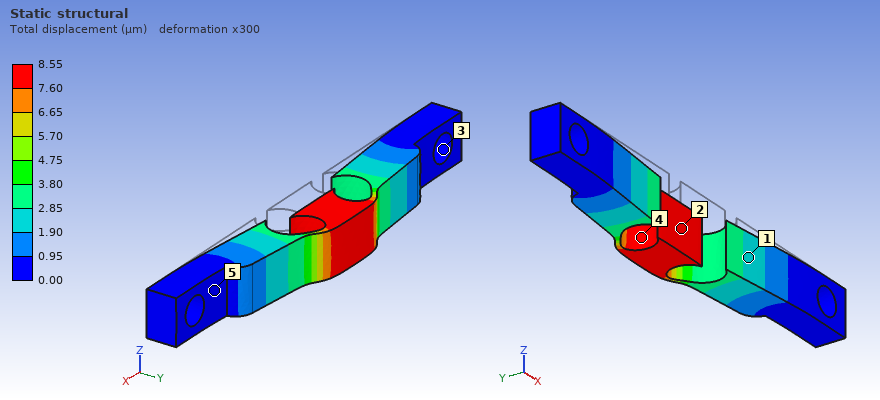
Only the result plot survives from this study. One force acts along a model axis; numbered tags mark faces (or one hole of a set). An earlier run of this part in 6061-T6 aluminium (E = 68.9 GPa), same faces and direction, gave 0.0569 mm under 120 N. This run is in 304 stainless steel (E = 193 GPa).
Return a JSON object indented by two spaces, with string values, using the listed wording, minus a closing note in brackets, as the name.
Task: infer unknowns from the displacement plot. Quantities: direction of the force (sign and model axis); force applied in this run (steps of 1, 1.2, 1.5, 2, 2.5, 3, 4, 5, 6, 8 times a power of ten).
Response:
{
  "direction of the force": "+Y",
  "force applied in this run": "50 N"
}
